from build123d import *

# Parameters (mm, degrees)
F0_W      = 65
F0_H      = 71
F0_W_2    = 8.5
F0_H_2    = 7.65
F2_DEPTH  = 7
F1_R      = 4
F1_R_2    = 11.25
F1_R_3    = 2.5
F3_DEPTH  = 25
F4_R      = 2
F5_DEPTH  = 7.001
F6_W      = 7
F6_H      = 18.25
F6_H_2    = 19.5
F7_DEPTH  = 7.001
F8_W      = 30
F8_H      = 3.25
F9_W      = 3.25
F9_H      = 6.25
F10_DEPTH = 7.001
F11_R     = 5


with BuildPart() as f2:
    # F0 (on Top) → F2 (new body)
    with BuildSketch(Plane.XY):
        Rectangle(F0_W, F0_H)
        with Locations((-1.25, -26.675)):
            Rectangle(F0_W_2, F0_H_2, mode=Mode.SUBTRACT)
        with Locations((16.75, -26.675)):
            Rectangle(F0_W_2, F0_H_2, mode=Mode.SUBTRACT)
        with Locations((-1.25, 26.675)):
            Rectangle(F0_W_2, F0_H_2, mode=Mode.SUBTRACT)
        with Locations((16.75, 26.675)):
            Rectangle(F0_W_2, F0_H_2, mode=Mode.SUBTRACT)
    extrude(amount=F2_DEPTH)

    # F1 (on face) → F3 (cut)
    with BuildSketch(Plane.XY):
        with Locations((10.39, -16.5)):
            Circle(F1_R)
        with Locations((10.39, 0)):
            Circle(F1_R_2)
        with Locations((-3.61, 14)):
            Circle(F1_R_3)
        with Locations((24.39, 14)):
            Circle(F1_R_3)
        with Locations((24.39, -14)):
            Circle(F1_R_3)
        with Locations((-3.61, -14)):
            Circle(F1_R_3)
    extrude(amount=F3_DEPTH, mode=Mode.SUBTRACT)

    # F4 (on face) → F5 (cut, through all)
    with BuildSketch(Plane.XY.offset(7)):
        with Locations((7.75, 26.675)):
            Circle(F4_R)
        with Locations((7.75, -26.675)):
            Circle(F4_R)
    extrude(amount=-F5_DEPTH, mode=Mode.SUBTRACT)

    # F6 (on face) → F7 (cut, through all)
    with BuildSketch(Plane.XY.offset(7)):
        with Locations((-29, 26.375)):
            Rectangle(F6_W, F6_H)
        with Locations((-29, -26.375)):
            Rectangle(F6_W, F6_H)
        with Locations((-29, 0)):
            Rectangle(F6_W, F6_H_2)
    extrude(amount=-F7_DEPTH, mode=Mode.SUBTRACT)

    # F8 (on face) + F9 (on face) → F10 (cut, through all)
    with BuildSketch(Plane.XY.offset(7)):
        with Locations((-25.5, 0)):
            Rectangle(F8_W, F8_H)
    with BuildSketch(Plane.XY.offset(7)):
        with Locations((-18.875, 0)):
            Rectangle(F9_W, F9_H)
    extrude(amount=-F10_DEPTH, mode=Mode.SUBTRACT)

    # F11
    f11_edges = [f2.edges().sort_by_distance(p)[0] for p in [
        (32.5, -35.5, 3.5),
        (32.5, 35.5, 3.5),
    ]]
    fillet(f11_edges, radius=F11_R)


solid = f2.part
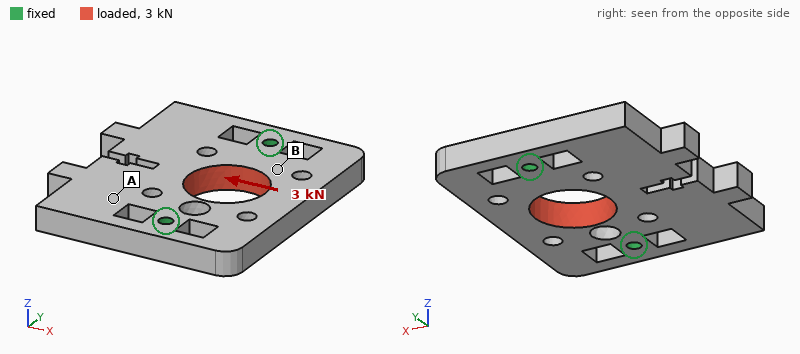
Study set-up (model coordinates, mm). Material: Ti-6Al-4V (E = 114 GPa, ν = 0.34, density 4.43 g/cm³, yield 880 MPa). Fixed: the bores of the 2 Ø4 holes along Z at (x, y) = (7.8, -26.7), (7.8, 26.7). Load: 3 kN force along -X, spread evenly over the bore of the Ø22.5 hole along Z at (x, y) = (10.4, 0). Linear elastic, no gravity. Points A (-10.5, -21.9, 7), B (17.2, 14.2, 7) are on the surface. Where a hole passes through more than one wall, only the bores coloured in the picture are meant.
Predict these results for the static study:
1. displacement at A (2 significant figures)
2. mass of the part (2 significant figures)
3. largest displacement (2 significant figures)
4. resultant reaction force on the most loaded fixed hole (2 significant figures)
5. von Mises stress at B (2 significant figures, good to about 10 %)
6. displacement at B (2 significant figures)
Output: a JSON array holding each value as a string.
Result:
["3.1 µm", "100 g", "9.0 µm", "1.5 kN", "16 MPa", "5.1 µm"]
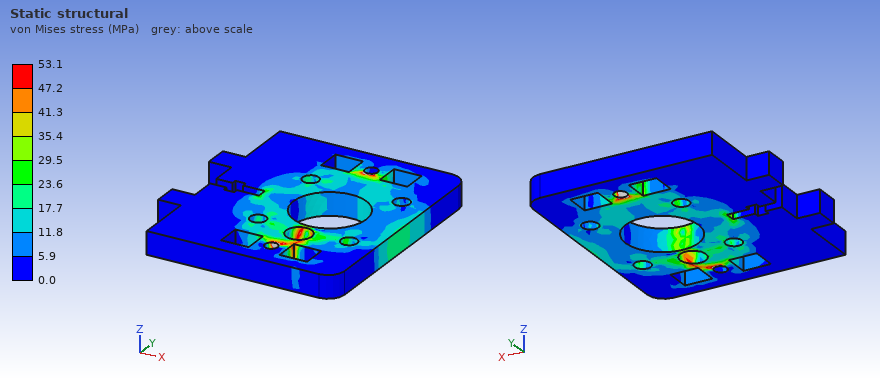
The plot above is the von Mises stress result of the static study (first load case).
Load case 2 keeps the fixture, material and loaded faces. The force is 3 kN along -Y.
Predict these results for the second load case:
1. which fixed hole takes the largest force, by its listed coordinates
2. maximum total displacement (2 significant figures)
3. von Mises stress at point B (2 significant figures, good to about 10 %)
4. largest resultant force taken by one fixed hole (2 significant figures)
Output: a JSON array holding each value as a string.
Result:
["(7.8, 26.7)", "6.1 µm", "13 MPa", "1.7 kN"]
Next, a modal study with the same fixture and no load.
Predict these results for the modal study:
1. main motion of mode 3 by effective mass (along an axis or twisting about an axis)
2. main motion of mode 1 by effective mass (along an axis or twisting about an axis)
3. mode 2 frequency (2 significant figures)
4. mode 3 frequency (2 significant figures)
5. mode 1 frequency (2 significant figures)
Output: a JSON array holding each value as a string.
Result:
["along Z", "along Z", "4400 Hz", "5000 Hz", "2600 Hz"]
